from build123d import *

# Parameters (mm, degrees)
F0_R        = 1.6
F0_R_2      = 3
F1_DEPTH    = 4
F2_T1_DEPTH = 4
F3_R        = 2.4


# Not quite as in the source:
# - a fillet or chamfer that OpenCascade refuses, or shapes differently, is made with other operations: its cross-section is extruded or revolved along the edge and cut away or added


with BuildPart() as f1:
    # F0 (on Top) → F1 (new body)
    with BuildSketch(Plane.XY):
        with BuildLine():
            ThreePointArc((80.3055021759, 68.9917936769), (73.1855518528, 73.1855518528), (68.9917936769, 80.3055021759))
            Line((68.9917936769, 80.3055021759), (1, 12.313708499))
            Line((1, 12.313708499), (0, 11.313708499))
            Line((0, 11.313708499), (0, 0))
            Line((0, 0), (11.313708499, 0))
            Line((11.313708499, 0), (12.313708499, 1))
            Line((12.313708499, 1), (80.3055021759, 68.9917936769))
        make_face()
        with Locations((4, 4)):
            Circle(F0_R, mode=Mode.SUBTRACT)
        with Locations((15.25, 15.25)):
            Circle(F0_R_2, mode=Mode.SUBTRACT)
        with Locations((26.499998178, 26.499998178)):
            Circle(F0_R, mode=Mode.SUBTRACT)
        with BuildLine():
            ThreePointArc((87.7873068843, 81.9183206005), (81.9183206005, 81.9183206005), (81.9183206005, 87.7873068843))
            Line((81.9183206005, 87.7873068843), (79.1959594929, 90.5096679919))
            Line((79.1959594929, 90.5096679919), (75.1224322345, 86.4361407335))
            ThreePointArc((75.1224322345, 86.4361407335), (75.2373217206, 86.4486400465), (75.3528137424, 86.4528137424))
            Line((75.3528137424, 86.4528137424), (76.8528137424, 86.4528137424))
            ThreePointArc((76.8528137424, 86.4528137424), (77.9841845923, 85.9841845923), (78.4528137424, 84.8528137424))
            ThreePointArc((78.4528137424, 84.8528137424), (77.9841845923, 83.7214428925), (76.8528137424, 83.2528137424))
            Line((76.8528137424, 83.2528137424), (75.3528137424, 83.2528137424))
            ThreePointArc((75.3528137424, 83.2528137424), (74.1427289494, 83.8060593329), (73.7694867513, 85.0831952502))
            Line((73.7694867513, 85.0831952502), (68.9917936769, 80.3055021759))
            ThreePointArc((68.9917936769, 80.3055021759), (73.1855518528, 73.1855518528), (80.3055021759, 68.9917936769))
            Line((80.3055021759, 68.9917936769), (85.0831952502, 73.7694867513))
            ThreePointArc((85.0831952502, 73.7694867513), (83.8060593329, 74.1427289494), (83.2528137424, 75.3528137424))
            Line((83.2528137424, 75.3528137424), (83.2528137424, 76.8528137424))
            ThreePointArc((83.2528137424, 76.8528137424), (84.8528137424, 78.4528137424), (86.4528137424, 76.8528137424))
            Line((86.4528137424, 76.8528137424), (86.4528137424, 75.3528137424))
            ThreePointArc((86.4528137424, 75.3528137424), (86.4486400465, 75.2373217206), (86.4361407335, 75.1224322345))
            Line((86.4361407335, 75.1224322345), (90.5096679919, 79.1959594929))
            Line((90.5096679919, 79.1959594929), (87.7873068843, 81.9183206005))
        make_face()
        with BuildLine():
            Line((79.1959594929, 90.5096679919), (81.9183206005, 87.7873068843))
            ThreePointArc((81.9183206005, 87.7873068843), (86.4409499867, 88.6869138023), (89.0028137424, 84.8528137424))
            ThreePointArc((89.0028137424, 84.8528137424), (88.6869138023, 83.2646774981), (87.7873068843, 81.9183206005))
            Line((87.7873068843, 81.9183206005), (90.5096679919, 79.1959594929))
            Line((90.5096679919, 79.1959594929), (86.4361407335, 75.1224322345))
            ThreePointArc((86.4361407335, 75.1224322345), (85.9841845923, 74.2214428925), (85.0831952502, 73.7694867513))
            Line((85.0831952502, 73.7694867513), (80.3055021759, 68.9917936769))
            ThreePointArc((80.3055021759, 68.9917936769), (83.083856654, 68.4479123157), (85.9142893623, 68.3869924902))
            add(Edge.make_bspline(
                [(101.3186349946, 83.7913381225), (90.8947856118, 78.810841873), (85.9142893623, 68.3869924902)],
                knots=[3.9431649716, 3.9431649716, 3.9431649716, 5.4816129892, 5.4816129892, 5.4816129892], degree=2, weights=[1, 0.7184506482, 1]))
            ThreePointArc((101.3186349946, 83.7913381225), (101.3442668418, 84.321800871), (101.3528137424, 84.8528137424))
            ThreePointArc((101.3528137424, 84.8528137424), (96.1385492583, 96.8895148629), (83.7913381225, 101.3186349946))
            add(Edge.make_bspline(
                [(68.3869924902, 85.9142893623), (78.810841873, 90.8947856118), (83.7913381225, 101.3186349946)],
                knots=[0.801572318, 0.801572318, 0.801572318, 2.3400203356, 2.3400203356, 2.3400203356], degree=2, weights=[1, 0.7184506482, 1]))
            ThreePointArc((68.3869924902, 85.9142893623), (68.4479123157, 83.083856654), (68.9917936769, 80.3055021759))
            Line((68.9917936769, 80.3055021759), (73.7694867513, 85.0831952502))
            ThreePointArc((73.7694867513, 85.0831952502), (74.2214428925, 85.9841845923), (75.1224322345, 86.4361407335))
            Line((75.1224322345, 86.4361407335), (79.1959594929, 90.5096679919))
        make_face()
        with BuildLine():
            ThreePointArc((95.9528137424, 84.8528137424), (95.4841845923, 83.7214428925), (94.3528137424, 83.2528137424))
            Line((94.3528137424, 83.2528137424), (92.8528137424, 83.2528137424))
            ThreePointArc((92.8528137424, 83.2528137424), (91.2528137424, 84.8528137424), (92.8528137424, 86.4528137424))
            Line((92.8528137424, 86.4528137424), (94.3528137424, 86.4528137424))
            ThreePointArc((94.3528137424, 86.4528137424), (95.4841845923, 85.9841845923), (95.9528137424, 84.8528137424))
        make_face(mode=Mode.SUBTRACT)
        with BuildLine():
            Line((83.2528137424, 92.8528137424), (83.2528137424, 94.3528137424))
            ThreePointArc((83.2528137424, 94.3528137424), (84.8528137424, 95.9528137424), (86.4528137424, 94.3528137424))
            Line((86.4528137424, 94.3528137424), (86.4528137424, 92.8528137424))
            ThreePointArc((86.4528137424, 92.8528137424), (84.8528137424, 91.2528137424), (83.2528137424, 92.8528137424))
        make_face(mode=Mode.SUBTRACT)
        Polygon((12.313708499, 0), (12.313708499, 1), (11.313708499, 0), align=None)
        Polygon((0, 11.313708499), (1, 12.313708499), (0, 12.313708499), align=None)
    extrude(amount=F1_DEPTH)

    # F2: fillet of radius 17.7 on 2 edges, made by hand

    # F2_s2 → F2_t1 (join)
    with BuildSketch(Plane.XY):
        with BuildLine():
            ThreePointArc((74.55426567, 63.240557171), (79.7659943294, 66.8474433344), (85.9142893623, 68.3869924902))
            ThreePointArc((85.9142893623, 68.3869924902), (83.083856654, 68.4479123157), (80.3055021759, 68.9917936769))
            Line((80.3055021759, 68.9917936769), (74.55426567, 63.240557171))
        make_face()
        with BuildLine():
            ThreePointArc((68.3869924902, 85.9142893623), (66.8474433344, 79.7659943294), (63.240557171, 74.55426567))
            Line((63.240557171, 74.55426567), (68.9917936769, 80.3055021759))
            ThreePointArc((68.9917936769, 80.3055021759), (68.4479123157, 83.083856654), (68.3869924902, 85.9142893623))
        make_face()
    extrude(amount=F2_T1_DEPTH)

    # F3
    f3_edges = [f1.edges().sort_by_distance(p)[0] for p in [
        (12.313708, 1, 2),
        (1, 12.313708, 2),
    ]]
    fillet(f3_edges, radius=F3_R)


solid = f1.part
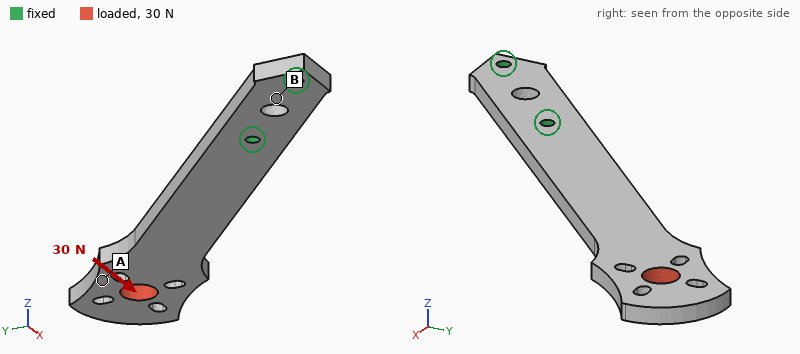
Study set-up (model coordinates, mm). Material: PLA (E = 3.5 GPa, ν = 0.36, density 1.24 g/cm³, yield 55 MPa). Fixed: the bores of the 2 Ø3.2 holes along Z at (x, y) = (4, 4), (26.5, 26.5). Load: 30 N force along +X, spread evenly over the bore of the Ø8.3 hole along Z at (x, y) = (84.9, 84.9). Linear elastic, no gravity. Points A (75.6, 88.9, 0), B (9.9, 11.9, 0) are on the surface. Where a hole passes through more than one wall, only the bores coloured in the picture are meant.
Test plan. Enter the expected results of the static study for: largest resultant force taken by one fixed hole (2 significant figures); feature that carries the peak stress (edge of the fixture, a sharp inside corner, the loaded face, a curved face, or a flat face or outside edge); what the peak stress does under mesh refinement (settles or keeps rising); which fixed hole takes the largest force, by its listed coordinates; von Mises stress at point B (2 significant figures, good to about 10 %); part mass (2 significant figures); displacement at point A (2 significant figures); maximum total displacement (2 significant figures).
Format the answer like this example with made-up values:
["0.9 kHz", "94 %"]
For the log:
["63 N", "edge of the fixture", "keeps rising", "(26.5, 26.5)", "2.2 MPa", "11 g", "1.1 mm", "1.4 mm"]
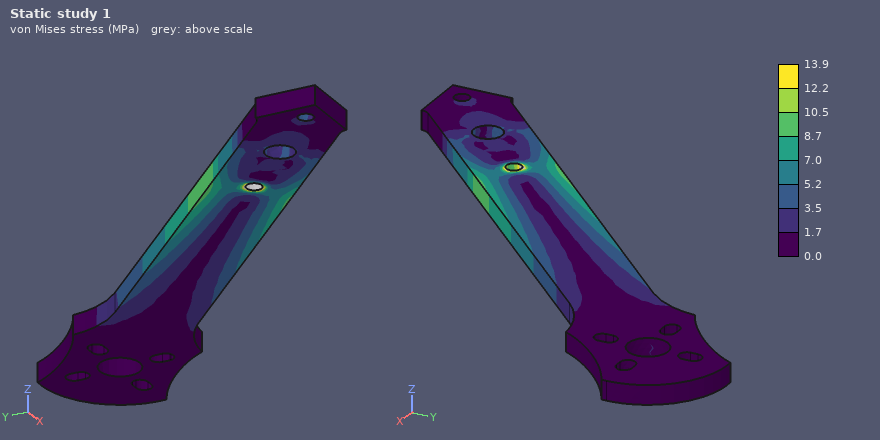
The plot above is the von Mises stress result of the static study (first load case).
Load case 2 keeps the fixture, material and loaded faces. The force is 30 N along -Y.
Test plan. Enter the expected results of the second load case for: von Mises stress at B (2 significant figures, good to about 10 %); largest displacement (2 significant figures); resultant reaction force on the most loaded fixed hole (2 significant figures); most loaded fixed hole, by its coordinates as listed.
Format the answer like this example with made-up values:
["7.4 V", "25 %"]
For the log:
["2.1 MPa", "1.4 mm", "63 N", "(26.5, 26.5)"]
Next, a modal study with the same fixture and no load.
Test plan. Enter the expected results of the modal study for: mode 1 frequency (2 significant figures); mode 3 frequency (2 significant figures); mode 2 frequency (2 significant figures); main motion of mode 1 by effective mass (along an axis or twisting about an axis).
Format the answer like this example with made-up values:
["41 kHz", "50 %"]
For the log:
["110 Hz", "680 Hz", "350 Hz", "along Z"]
